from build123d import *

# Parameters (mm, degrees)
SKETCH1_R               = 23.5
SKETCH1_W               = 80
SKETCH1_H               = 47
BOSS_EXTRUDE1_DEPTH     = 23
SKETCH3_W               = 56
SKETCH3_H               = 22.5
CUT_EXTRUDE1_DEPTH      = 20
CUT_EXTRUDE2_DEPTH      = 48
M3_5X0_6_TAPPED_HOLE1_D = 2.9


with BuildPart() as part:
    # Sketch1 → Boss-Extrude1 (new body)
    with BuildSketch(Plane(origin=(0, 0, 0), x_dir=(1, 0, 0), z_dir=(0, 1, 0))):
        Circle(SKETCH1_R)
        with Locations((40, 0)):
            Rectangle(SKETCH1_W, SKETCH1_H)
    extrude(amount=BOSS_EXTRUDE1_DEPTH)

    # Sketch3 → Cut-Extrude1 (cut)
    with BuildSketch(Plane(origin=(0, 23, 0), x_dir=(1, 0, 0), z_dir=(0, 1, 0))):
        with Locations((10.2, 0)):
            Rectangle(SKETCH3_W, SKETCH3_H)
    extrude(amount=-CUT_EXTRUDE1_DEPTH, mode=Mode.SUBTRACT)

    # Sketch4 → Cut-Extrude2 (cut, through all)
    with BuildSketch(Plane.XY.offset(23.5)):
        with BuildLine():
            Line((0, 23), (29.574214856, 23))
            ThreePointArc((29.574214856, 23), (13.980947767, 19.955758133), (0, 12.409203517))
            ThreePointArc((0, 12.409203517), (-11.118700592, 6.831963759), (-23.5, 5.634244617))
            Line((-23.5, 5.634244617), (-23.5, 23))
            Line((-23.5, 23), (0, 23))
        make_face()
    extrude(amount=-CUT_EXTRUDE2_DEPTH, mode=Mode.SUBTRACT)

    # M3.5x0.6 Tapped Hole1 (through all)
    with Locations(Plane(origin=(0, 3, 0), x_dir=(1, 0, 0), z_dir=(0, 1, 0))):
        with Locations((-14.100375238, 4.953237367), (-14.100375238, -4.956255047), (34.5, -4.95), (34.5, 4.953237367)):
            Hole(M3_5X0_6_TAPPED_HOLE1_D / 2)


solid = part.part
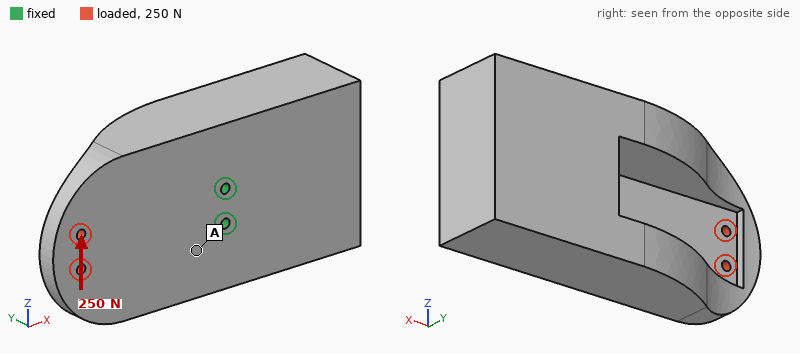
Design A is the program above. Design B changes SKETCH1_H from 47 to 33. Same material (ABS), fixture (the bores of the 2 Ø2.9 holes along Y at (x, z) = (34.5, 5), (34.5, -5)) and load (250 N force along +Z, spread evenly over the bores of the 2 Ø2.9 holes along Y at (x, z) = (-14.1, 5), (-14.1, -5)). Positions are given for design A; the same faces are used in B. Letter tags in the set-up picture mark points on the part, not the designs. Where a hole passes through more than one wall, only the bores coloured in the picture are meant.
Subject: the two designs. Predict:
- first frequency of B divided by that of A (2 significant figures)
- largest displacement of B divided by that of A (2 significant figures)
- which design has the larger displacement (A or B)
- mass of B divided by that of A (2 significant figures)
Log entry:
1.1
1.1
B
0.70
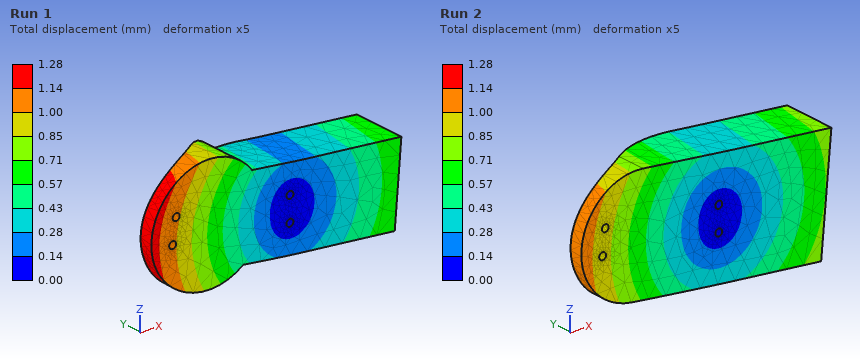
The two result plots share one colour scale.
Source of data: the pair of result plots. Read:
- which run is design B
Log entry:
Run 1
